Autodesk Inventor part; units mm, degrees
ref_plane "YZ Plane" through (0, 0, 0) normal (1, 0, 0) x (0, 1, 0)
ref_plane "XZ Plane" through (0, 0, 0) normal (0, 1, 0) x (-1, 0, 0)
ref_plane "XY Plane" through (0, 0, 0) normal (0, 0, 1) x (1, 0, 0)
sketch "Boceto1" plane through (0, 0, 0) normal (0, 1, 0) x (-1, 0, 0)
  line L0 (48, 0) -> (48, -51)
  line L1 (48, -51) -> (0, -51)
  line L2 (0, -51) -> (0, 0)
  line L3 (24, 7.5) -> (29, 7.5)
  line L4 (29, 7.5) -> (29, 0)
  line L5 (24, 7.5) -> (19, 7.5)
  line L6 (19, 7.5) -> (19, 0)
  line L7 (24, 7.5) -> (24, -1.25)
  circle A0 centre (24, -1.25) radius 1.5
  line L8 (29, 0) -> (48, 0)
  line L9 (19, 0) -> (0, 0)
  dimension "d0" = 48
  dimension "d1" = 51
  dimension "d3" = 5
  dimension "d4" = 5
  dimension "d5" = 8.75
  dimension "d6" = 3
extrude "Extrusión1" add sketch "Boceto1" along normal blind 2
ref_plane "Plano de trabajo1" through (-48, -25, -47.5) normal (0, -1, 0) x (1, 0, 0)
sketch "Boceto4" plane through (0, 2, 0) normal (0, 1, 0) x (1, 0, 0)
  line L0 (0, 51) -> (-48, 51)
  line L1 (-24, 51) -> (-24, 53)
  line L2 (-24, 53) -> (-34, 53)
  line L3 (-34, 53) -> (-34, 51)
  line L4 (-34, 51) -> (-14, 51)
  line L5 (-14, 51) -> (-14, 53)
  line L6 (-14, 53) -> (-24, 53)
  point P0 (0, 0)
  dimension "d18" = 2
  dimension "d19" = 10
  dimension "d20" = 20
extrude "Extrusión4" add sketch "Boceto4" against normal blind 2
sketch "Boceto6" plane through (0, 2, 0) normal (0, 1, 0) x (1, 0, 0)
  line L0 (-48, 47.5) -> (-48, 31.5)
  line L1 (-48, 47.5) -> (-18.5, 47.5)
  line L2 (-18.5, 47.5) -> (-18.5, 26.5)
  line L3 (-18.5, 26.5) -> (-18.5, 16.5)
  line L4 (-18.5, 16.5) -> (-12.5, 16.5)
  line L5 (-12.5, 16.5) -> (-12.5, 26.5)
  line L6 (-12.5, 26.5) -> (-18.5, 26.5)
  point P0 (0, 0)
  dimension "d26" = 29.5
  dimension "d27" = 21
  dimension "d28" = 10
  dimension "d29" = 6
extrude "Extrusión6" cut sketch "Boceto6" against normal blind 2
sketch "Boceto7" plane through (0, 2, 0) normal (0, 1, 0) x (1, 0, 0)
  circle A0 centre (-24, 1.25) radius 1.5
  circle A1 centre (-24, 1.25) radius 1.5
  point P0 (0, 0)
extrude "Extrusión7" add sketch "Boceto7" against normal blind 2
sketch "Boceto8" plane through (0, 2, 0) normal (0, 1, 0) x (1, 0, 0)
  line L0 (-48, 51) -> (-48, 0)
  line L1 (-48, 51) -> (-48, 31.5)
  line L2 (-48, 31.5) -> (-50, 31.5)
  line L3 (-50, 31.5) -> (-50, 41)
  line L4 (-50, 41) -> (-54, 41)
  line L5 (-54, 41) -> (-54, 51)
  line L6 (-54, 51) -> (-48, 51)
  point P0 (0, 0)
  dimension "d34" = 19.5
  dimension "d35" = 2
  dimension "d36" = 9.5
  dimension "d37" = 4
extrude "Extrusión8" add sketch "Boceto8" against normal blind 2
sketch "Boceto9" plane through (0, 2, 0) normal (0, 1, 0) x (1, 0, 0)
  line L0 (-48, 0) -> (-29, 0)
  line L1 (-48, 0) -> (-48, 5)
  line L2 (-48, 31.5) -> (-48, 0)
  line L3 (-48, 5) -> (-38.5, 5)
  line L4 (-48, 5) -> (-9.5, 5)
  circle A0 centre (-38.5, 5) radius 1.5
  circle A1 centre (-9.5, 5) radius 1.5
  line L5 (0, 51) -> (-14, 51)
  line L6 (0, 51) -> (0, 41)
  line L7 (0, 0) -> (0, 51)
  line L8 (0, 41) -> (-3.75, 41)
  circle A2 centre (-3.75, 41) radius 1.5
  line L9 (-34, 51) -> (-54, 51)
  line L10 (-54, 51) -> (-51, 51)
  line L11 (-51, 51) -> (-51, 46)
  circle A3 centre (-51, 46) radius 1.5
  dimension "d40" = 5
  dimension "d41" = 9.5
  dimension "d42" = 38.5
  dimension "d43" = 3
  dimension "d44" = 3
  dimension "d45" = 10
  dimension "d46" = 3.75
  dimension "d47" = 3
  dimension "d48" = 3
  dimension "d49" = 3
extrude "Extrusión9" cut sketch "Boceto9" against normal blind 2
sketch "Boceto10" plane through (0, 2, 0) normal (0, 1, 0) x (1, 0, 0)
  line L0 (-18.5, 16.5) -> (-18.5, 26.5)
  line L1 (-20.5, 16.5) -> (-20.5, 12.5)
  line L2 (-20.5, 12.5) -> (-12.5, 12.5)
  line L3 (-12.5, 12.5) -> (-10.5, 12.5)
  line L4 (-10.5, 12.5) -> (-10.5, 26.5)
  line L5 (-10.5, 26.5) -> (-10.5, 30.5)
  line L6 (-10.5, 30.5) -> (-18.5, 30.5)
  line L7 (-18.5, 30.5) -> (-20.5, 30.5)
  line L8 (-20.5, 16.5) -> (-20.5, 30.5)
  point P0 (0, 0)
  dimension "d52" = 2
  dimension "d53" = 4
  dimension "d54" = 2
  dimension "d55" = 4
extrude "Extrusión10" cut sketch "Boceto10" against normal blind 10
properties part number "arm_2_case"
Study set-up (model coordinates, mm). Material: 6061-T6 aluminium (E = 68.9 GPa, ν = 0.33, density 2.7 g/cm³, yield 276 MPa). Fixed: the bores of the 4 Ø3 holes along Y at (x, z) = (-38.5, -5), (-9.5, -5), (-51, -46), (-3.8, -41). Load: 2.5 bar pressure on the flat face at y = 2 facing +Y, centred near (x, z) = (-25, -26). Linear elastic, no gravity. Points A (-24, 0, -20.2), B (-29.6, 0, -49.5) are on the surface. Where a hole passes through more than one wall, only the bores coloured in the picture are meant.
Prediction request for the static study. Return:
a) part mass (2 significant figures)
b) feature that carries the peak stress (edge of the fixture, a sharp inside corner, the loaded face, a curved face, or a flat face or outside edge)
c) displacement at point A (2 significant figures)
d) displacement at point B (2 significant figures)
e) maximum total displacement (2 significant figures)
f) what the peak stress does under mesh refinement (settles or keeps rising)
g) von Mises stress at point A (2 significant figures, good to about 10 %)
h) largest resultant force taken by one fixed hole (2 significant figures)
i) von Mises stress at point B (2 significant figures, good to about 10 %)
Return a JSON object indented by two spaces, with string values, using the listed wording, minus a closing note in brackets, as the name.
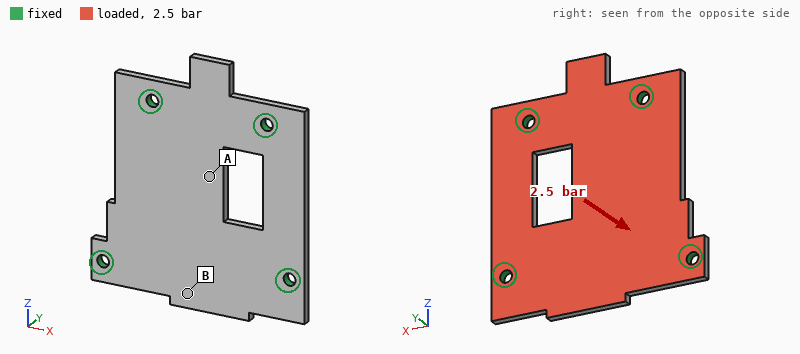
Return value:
{
  "part mass": "13 g",
  "feature that carries the peak stress": "edge of the fixture",
  "displacement at point A": "65 µm",
  "displacement at point B": "84 µm",
  "maximum total displacement": "89 µm",
  "what the peak stress does under mesh refinement": "keeps rising",
  "von Mises stress at point A": "17 MPa",
  "largest resultant force taken by one fixed hole": "180 N",
  "von Mises stress at point B": "36 MPa"
}
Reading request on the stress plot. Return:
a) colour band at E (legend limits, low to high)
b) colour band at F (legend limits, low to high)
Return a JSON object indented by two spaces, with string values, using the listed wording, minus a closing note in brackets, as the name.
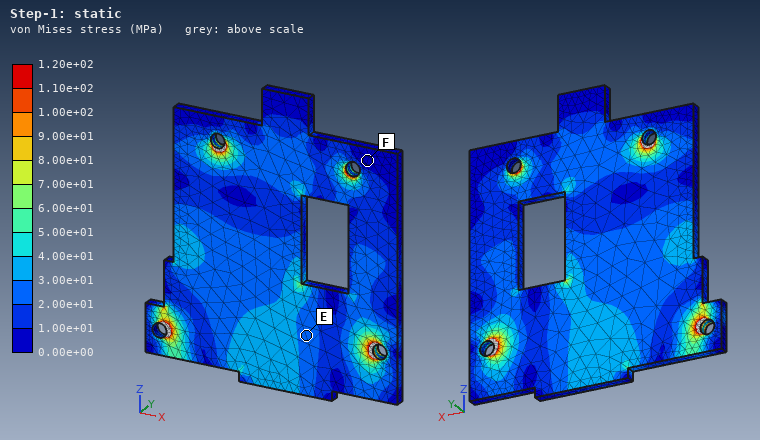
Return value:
{
  "colour band at E": "2.00e+01 to 3.00e+01 MPa",
  "colour band at F": "0.00e+00 to 1.00e+01 MPa"
}
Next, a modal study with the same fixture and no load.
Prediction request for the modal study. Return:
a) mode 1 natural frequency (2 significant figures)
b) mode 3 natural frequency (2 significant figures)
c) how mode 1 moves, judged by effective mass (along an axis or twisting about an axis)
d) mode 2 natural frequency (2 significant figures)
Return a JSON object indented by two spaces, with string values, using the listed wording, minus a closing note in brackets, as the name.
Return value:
{
  "mode 1 natural frequency": "4200 Hz",
  "mode 3 natural frequency": "7700 Hz",
  "how mode 1 moves, judged by effective mass": "along Y",
  "mode 2 natural frequency": "5700 Hz"
}
